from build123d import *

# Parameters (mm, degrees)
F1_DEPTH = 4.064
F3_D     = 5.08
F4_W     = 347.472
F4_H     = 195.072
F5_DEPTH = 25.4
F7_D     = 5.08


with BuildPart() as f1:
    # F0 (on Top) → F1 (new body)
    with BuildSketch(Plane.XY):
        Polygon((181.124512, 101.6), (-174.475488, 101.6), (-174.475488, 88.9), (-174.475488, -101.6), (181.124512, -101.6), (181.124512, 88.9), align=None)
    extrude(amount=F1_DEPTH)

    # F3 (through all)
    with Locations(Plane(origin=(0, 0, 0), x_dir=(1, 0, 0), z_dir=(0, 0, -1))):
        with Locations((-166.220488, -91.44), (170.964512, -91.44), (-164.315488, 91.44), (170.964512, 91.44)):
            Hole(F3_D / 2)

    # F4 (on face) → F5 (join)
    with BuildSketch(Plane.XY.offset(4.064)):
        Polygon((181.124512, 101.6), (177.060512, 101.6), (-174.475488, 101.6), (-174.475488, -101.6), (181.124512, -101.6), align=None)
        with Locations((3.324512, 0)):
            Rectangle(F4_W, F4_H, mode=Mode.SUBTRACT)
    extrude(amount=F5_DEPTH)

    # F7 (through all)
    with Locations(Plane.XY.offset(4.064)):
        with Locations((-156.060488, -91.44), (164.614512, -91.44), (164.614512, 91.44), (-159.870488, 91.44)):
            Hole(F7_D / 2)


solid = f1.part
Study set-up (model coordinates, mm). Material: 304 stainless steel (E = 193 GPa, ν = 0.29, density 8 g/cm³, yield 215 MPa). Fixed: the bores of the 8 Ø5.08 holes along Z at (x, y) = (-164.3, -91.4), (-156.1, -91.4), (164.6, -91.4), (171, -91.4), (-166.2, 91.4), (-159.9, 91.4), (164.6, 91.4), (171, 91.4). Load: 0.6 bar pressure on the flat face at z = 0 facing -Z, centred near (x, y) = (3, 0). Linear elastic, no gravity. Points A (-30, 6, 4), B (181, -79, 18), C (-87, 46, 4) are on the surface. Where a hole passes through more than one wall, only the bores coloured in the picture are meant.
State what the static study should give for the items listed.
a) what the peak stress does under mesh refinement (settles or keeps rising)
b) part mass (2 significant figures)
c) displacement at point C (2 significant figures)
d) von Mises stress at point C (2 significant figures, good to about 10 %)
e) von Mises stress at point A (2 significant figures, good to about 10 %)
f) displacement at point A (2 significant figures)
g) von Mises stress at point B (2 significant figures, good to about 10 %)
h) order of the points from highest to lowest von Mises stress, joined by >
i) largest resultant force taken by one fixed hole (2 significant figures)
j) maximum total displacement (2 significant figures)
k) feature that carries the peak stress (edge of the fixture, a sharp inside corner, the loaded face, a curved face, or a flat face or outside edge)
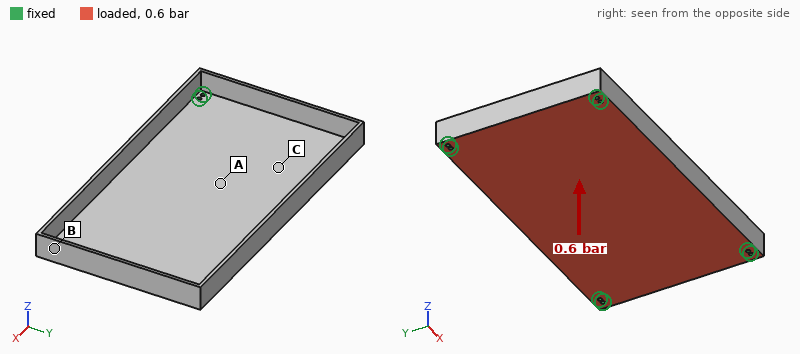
keeps rising
3.3 kg
0.36 mm
35 MPa
53 MPa
0.63 mm
25 MPa
A > C > B
2.3 kN
0.66 mm
edge of the fixture
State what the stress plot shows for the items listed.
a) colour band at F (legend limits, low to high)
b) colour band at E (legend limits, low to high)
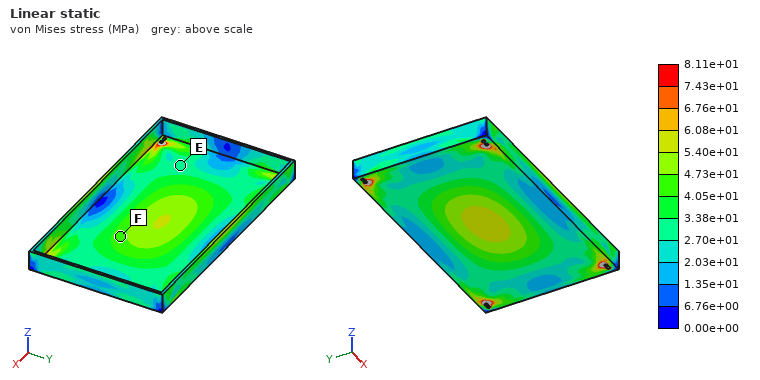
4.05e+01 to 4.73e+01 MPa
2.70e+01 to 3.38e+01 MPa
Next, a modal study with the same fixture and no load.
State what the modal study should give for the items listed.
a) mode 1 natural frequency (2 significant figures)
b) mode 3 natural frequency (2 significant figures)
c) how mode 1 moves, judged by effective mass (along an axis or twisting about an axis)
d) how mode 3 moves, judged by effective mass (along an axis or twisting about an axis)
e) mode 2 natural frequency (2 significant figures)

330 Hz
740 Hz
along Z
twisting about X
610 Hz
